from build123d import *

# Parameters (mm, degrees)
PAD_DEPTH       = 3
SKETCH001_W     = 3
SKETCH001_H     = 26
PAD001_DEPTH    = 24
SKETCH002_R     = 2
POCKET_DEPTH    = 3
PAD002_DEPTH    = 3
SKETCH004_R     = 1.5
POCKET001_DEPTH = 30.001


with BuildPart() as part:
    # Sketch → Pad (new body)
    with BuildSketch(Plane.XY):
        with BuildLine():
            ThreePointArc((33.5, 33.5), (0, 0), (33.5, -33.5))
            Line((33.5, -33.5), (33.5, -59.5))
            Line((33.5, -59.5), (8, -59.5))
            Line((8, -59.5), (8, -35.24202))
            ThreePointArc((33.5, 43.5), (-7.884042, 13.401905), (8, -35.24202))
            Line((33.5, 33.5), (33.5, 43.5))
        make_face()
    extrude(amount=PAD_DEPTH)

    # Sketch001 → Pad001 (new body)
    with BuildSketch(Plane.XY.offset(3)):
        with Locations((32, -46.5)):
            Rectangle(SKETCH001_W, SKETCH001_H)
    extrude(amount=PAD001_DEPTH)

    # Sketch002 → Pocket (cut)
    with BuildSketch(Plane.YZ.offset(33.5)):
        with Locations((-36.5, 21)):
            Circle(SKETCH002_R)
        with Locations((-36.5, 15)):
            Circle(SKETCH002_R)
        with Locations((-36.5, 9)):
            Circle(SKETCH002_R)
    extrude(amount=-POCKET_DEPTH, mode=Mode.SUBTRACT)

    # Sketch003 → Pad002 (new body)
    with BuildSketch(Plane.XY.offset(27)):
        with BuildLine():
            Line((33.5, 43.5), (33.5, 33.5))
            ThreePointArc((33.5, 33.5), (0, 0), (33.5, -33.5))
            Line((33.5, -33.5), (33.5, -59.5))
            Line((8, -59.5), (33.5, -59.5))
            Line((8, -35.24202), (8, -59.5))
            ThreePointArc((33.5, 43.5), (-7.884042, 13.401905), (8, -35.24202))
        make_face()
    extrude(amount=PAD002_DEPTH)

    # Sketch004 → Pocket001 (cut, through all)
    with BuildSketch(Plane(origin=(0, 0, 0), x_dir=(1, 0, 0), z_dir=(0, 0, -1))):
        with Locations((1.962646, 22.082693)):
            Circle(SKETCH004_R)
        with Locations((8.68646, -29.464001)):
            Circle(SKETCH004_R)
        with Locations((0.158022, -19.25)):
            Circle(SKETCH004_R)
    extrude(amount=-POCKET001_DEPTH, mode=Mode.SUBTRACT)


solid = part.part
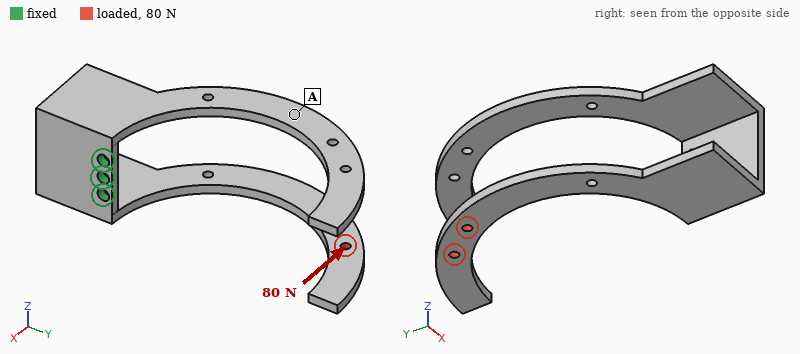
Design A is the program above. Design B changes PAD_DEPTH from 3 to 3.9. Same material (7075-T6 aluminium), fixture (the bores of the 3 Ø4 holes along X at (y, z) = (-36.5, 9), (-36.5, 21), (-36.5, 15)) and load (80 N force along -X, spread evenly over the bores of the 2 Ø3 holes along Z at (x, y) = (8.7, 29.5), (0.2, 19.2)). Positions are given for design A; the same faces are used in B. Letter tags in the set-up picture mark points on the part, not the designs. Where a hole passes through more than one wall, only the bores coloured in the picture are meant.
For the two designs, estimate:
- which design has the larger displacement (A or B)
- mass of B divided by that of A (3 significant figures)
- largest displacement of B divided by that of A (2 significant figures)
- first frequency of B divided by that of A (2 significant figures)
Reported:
A
1.12
0.80
1.0
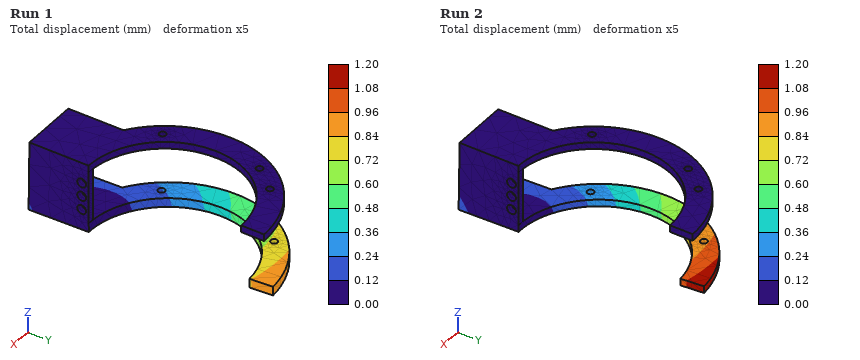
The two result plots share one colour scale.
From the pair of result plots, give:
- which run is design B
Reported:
Run 1
